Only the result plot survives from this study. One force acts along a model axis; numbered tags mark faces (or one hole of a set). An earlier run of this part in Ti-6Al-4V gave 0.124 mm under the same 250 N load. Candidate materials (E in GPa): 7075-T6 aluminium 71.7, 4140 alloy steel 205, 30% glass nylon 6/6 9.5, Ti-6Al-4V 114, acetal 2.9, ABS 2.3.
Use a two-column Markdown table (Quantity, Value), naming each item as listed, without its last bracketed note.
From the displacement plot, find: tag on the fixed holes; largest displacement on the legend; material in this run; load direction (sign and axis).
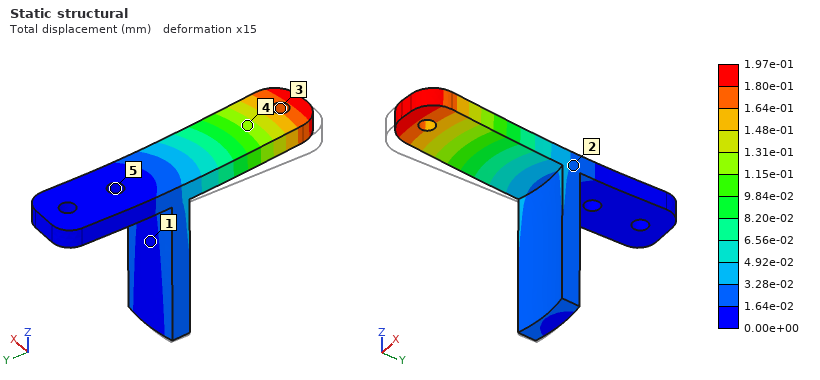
| Quantity | Value |
|---|---|
| tag on the fixed holes | 5 |
| largest displacement on the legend | 1.97e-01 mm |
| material in this run | 7075-T6 aluminium |
| load direction | +X |
